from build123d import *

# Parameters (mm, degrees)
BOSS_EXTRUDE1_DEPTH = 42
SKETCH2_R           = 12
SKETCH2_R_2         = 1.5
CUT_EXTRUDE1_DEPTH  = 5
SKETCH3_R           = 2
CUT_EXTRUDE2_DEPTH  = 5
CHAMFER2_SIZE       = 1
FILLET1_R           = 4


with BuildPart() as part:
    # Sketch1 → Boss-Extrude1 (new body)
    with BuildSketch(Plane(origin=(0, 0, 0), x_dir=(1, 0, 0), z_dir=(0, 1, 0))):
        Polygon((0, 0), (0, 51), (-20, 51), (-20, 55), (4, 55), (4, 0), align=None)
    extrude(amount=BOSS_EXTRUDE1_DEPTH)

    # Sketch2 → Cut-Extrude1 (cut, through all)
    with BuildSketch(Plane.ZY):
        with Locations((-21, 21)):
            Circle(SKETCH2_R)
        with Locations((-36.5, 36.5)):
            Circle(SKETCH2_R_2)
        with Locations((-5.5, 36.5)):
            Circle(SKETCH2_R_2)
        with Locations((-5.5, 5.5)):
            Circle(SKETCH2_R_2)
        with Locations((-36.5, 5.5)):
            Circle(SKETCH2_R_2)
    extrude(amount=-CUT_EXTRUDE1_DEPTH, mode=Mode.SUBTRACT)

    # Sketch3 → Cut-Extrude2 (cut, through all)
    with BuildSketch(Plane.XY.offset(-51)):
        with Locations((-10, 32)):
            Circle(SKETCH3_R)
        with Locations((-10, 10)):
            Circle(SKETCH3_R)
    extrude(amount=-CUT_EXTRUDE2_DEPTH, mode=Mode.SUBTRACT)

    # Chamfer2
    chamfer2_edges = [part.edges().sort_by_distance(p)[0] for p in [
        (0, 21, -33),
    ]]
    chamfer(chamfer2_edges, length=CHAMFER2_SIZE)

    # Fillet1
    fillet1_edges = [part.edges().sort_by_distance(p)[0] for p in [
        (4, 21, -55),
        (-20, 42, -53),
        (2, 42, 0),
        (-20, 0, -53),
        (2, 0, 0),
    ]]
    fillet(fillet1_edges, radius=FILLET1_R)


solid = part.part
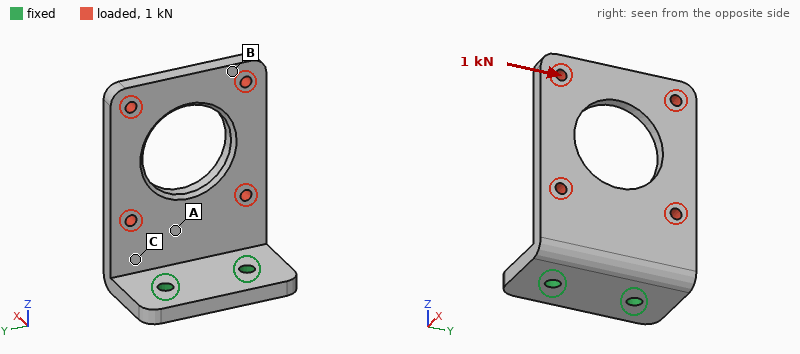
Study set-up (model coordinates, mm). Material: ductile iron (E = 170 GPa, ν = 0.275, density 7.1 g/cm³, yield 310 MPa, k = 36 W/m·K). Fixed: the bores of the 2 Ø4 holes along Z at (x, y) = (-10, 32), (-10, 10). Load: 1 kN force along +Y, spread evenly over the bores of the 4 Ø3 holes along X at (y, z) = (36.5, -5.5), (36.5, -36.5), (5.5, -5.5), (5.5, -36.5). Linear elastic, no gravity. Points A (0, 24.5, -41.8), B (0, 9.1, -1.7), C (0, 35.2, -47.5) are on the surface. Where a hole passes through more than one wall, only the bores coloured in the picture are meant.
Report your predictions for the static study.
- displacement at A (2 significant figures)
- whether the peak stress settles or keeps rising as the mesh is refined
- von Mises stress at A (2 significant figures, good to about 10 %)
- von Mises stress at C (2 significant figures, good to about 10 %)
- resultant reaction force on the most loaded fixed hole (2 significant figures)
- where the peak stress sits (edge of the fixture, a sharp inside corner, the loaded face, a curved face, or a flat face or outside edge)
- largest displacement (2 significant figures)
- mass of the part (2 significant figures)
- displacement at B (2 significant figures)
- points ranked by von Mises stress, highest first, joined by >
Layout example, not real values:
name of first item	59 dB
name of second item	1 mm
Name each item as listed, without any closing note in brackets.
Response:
displacement at A	0.026 mm
whether the peak stress settles or keeps rising as the mesh is refined	keeps rising
von Mises stress at A	49 MPa
von Mises stress at C	72 MPa
resultant reaction force on the most loaded fixed hole	1.4 kN
where the peak stress sits	edge of the fixture
largest displacement	0.13 mm
mass of the part	73 g
displacement at B	0.12 mm
points ranked by von Mises stress, highest first, joined by >	C > A > B
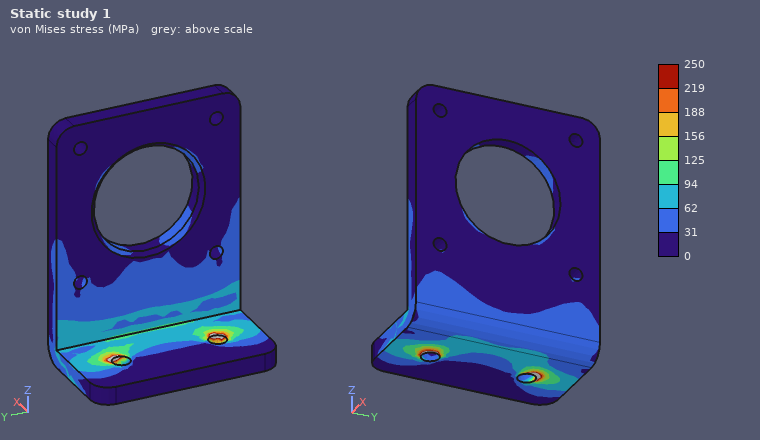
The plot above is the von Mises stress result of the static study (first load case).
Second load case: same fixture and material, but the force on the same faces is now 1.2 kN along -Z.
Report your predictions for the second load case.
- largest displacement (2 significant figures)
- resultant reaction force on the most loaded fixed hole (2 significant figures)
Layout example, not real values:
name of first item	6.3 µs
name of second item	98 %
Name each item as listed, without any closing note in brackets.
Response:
largest displacement	0.13 mm
resultant reaction force on the most loaded fixed hole	600 N
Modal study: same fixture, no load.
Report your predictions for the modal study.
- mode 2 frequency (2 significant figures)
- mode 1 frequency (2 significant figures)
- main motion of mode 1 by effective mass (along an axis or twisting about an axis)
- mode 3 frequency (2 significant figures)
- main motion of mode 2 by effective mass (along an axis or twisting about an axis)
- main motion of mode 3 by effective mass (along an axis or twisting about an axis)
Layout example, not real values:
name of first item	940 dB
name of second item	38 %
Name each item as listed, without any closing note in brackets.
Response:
mode 2 frequency	2400 Hz
mode 1 frequency	900 Hz
main motion of mode 1 by effective mass	along X
mode 3 frequency	3100 Hz
main motion of mode 2 by effective mass	along Y
main motion of mode 3 by effective mass	along Y
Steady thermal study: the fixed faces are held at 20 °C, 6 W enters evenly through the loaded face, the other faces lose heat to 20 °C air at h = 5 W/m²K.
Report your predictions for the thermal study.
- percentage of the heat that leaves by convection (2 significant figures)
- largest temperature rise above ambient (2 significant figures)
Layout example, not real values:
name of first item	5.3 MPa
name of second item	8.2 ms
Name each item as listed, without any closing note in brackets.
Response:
percentage of the heat that leaves by convection	13 %
largest temperature rise above ambient	54 K
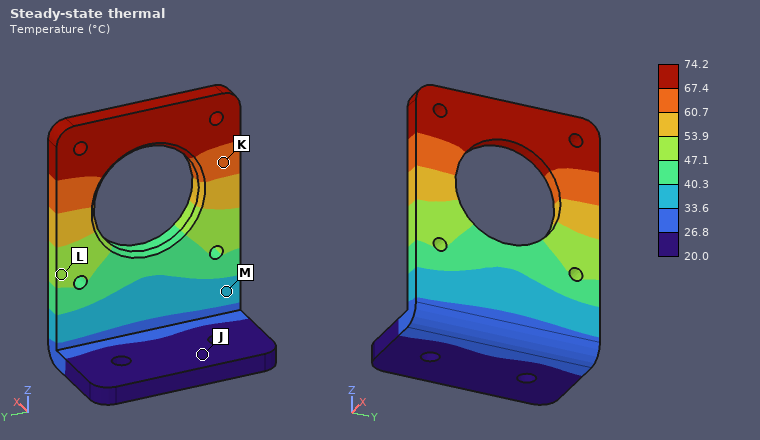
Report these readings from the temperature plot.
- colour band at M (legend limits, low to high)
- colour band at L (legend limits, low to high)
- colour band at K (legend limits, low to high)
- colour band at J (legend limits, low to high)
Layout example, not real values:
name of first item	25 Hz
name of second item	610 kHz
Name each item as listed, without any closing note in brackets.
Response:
colour band at M	33.6 to 40.3 °C
colour band at L	47.1 to 53.9 °C
colour band at K	60.7 to 67.4 °C
colour band at J	20.0 to 26.8 °C
